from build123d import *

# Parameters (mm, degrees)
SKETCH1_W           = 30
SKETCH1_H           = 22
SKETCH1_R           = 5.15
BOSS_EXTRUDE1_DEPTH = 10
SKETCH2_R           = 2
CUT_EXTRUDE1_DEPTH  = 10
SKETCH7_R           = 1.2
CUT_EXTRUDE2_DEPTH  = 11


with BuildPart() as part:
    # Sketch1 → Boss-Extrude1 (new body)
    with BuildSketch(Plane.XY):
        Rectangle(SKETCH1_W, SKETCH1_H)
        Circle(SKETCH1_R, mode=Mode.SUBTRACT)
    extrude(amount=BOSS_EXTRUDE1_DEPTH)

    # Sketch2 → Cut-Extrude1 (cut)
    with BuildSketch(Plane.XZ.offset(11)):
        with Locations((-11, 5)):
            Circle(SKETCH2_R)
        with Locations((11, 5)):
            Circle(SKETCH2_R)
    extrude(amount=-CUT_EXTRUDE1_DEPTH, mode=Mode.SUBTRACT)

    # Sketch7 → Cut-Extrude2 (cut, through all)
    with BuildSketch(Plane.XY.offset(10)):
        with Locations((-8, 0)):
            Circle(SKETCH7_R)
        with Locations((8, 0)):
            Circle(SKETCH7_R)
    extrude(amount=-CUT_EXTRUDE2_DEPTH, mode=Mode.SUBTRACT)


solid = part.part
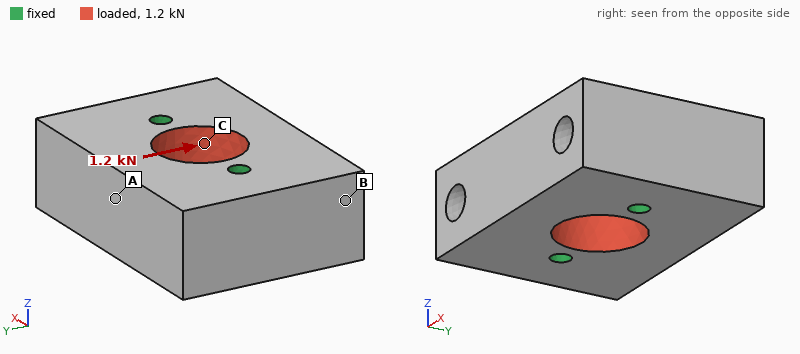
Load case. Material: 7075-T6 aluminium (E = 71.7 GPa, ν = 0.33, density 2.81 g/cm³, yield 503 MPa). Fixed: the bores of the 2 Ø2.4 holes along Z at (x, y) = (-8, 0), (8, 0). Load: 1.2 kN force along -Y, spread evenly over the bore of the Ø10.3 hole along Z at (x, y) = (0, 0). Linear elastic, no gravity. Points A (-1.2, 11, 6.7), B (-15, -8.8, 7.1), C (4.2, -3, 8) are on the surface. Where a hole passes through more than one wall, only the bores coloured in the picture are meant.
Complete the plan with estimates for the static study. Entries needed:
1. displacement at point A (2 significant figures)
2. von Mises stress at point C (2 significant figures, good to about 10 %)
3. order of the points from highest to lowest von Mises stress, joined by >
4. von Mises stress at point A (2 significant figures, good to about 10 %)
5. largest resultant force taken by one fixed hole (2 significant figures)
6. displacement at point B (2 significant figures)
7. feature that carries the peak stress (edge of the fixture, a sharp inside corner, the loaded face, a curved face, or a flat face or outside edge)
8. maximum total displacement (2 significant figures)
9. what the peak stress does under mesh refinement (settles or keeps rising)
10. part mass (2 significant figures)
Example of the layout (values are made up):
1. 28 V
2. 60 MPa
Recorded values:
1. 0.80 µm
2. 9.2 MPa
3. C > A > B
4. 5.4 MPa
5. 600 N
6. 0.19 µm
7. edge of the fixture
8. 1.1 µm
9. keeps rising
10. 15 g
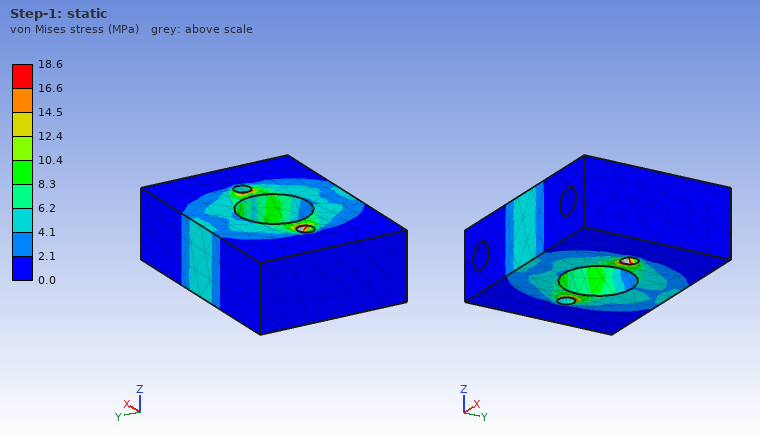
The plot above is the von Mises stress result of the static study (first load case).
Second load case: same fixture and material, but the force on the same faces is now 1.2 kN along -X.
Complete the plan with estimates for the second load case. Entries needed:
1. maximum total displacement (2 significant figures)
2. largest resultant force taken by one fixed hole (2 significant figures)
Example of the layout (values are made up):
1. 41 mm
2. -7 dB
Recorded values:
1. 1.0 µm
2. 600 N
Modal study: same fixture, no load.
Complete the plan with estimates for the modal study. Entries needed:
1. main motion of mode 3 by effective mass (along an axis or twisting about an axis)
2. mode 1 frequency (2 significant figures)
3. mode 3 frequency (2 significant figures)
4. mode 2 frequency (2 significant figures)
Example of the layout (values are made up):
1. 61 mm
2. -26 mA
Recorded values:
1. along Z
2. 32 kHz
3. 38 kHz
4. 33 kHz
